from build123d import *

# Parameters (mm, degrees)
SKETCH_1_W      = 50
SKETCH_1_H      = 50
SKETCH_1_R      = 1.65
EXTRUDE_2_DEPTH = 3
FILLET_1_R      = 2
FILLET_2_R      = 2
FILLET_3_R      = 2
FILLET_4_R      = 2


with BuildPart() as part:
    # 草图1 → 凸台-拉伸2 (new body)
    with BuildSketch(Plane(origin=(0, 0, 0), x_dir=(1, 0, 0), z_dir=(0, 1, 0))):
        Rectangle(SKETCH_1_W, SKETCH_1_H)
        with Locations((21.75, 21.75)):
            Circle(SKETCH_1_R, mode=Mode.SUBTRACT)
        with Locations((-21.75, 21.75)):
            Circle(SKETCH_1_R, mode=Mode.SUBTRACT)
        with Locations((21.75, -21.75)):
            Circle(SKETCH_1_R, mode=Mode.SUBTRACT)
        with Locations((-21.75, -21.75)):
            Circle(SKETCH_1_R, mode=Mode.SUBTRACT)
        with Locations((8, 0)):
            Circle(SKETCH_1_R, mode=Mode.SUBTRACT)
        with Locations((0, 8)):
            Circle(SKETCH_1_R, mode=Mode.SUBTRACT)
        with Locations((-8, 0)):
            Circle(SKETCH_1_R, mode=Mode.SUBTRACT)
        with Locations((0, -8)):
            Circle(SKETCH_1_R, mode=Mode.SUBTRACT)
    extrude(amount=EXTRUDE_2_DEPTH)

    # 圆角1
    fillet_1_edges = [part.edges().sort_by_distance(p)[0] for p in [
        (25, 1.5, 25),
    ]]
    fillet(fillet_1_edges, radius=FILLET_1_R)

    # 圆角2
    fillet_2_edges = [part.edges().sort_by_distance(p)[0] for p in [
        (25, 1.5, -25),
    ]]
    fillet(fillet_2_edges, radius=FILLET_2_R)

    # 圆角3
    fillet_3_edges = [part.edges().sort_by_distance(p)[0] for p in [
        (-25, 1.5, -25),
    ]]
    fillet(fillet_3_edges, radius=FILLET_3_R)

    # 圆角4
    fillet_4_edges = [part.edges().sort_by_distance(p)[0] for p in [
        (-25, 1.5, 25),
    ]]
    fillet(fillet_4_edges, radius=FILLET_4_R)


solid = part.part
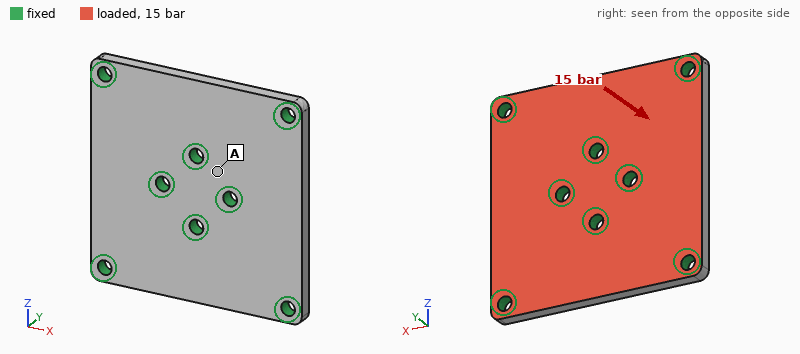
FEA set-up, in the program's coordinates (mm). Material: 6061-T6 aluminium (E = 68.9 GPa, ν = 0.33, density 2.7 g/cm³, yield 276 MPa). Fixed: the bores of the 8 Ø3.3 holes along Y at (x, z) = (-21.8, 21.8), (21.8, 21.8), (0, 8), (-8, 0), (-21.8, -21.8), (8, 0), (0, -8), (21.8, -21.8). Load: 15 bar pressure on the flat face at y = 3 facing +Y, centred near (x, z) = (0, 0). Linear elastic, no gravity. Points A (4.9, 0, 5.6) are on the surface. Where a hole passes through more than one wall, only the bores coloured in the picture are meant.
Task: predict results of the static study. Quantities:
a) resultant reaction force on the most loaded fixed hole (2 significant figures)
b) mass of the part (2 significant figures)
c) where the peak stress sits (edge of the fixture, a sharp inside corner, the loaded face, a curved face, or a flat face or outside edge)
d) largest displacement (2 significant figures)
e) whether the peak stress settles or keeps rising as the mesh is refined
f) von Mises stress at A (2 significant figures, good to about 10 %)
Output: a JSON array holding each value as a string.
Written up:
["500 N", "20 g", "edge of the fixture", "38 µm", "keeps rising", "21 MPa"]
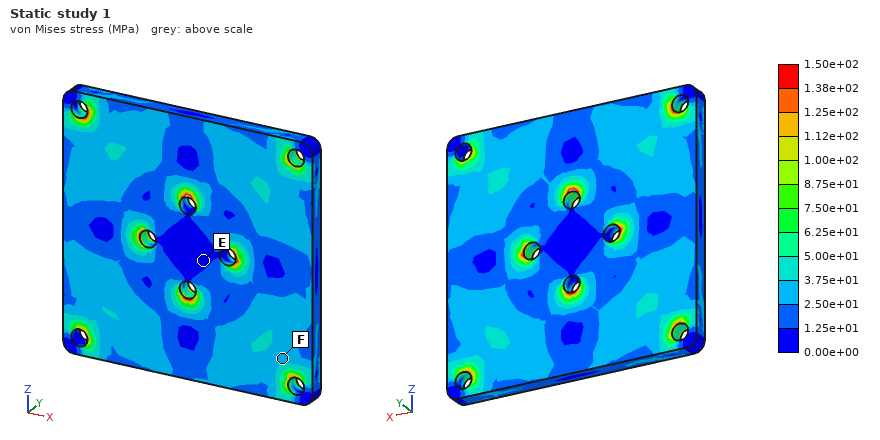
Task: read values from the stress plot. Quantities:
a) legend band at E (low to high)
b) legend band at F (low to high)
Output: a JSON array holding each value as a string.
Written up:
["0.00e+00 to 1.25e+01 MPa", "2.50e+01 to 3.75e+01 MPa"]
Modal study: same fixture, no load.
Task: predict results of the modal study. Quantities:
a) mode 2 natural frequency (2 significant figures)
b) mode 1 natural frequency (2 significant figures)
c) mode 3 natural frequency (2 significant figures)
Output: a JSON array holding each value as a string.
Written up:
["14 kHz", "13 kHz", "14 kHz"]
